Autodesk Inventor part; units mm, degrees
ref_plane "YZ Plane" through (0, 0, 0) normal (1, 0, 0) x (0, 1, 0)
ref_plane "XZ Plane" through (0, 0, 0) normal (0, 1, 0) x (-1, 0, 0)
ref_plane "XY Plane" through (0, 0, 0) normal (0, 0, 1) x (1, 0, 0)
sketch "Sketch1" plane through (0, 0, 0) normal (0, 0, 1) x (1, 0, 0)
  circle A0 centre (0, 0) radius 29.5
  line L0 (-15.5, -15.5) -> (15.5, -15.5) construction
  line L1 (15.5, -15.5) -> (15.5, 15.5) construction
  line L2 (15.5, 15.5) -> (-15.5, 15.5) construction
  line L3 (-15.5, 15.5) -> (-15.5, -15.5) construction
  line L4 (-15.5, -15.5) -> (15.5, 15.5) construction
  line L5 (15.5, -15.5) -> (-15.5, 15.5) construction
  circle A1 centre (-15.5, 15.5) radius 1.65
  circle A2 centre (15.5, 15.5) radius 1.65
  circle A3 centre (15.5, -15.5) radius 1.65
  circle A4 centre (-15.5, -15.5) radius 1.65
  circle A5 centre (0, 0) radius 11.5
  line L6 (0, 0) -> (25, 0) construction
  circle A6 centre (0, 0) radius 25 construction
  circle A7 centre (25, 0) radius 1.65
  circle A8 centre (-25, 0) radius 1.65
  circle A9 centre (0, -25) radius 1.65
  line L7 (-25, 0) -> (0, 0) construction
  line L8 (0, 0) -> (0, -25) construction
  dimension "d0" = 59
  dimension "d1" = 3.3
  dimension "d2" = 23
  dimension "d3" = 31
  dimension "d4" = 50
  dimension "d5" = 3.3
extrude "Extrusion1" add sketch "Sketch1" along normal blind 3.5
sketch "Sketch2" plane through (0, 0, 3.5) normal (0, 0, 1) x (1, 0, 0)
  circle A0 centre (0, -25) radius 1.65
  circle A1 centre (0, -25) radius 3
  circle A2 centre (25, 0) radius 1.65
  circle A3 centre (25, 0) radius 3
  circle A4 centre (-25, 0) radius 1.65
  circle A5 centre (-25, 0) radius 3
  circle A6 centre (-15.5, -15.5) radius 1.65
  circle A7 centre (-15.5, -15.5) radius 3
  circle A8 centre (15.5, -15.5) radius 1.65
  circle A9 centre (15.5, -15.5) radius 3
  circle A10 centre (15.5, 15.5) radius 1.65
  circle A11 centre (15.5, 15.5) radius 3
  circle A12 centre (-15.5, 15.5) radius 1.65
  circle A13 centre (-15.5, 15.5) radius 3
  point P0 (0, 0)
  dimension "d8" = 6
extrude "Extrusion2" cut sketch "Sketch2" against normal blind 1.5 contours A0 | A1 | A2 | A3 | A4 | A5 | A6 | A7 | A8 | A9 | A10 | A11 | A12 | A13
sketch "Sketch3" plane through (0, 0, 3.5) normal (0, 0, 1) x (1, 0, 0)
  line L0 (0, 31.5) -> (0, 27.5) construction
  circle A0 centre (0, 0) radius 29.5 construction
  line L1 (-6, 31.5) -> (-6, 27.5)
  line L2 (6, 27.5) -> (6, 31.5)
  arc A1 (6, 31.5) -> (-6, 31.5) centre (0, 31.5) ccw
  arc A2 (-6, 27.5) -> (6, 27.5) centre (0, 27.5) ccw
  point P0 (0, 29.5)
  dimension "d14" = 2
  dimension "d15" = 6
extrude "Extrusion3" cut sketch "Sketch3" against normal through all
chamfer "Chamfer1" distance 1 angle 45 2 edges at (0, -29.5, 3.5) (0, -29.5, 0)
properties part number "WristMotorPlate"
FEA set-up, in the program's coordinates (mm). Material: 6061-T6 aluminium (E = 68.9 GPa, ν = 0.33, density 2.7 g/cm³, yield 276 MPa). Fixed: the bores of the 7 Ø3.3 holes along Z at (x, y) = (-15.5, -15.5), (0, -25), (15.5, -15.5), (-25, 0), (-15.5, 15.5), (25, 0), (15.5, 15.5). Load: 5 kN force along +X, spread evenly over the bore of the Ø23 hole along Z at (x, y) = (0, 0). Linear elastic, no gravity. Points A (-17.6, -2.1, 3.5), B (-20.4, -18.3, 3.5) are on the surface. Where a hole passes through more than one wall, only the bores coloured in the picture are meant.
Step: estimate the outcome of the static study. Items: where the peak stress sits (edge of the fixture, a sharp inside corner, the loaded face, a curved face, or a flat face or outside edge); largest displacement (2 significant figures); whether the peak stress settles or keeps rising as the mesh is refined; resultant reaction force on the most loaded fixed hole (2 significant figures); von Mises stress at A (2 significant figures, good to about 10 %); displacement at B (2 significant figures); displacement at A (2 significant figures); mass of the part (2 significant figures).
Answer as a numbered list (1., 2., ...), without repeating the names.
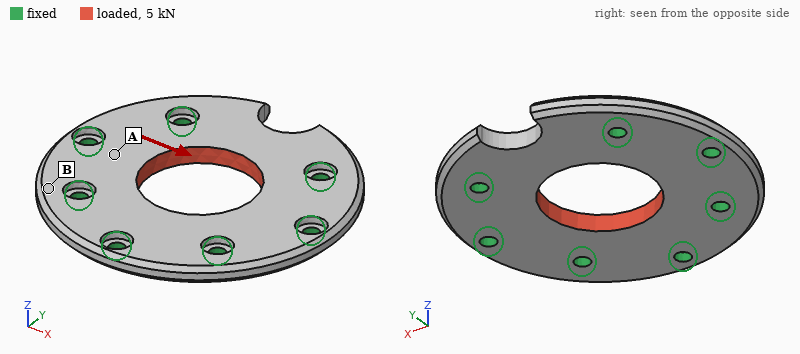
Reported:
1. edge of the fixture
2. 8.2 µm
3. keeps rising
4. 860 N
5. 20 MPa
6. 2.6 µm
7. 5.2 µm
8. 20 g
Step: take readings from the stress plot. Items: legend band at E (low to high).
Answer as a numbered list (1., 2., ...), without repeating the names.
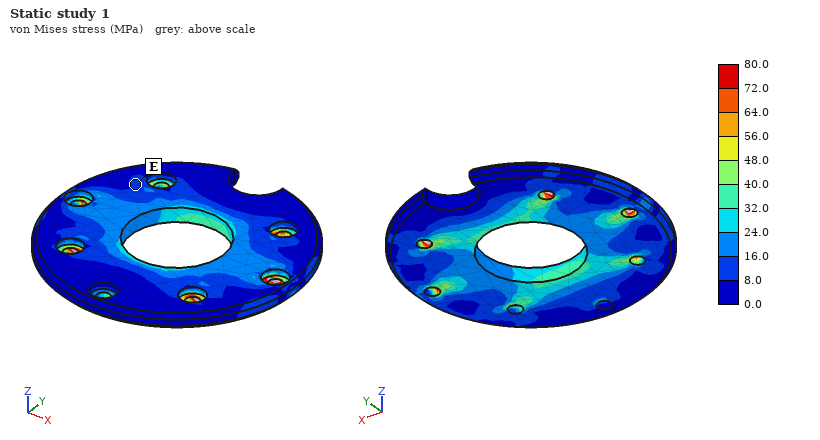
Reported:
1. 8.0 to 16.0 MPa
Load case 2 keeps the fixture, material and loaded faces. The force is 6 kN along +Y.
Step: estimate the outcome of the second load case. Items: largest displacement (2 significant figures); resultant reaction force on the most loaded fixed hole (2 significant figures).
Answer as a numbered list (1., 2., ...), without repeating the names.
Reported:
1. 17 µm
2. 1.3 kN
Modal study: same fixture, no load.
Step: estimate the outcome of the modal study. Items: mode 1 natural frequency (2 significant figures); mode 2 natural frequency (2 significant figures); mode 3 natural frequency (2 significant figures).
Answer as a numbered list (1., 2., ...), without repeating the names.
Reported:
1. 13 kHz
2. 17 kHz
3. 20 kHz
